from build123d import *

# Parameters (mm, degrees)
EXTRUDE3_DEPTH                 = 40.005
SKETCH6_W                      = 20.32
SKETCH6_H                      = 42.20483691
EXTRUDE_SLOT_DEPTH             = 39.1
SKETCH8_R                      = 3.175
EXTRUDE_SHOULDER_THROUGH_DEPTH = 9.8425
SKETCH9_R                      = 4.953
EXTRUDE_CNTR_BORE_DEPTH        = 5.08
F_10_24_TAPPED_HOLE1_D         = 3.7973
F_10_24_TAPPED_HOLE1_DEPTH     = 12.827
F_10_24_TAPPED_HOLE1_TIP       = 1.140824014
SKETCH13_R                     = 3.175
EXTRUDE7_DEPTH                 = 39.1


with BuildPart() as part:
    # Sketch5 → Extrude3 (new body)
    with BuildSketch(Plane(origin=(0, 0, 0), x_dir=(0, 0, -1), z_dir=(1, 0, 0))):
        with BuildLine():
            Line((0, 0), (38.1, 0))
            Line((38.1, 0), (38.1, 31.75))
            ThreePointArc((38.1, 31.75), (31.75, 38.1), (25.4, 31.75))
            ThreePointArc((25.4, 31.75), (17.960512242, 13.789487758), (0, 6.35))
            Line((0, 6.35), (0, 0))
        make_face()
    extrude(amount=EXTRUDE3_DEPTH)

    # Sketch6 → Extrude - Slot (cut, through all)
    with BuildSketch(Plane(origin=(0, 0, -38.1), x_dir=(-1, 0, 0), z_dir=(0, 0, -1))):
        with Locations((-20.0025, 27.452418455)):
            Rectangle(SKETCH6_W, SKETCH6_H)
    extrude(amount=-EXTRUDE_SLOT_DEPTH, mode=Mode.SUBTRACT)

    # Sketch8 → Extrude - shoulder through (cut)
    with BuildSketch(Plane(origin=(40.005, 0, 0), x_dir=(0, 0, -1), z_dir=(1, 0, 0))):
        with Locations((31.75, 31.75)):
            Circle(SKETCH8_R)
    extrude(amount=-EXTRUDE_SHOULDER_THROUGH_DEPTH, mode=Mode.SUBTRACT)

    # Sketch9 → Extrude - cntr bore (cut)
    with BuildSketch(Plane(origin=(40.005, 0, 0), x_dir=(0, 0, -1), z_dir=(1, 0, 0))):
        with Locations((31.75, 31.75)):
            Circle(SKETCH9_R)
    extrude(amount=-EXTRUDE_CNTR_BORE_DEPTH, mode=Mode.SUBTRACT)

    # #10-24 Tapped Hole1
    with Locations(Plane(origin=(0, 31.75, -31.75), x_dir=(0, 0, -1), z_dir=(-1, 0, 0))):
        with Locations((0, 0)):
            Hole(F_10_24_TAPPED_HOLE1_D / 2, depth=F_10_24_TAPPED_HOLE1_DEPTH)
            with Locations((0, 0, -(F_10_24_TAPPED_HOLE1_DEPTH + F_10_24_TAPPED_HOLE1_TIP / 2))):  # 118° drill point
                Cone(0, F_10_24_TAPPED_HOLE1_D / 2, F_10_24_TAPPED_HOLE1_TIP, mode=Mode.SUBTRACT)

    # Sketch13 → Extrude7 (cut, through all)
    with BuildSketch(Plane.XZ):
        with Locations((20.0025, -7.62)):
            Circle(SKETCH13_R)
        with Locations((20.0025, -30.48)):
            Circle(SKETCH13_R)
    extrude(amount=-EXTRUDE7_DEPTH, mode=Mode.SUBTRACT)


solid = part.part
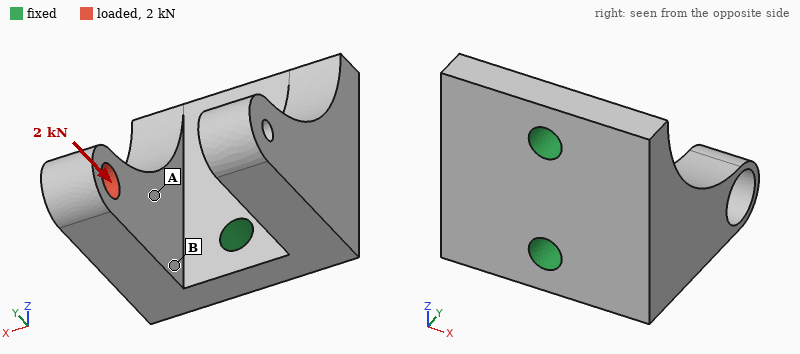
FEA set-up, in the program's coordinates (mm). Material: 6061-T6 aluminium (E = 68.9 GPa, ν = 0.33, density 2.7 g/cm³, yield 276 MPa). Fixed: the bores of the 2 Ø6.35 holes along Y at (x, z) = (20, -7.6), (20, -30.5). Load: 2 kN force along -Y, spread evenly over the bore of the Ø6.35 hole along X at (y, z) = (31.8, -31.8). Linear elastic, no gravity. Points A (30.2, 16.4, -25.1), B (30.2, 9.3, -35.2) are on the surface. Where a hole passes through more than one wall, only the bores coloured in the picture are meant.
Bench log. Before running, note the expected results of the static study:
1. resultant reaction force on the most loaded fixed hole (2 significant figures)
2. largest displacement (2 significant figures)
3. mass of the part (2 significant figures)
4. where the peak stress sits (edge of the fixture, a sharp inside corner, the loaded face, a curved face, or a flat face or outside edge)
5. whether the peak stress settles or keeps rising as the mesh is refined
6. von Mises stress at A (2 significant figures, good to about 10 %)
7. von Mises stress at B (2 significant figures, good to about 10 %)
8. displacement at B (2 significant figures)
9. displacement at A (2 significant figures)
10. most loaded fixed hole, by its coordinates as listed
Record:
1.9 kN
98 µm
51 g
edge of the fixture
keeps rising
24 MPa
50 MPa
37 µm
42 µm
(20, -30.5)
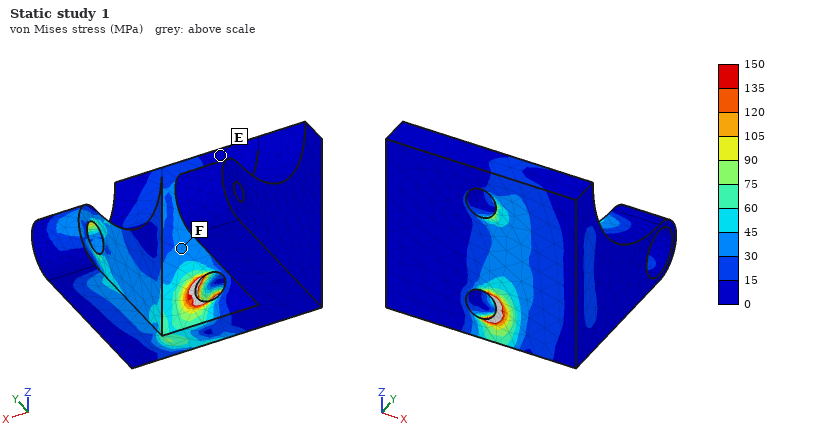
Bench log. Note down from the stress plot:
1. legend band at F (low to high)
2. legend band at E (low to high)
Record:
30 to 45 MPa
0 to 15 MPa
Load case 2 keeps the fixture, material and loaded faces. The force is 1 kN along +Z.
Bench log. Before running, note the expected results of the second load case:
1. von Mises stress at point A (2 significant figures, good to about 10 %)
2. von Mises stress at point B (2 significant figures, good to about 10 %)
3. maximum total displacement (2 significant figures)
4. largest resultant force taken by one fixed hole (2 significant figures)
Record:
31 MPa
40 MPa
0.11 mm
1.3 kN
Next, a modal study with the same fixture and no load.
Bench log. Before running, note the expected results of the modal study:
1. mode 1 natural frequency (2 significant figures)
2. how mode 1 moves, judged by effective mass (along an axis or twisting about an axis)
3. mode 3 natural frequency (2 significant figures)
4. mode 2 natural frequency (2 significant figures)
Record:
4000 Hz
along X
7800 Hz
4500 Hz
